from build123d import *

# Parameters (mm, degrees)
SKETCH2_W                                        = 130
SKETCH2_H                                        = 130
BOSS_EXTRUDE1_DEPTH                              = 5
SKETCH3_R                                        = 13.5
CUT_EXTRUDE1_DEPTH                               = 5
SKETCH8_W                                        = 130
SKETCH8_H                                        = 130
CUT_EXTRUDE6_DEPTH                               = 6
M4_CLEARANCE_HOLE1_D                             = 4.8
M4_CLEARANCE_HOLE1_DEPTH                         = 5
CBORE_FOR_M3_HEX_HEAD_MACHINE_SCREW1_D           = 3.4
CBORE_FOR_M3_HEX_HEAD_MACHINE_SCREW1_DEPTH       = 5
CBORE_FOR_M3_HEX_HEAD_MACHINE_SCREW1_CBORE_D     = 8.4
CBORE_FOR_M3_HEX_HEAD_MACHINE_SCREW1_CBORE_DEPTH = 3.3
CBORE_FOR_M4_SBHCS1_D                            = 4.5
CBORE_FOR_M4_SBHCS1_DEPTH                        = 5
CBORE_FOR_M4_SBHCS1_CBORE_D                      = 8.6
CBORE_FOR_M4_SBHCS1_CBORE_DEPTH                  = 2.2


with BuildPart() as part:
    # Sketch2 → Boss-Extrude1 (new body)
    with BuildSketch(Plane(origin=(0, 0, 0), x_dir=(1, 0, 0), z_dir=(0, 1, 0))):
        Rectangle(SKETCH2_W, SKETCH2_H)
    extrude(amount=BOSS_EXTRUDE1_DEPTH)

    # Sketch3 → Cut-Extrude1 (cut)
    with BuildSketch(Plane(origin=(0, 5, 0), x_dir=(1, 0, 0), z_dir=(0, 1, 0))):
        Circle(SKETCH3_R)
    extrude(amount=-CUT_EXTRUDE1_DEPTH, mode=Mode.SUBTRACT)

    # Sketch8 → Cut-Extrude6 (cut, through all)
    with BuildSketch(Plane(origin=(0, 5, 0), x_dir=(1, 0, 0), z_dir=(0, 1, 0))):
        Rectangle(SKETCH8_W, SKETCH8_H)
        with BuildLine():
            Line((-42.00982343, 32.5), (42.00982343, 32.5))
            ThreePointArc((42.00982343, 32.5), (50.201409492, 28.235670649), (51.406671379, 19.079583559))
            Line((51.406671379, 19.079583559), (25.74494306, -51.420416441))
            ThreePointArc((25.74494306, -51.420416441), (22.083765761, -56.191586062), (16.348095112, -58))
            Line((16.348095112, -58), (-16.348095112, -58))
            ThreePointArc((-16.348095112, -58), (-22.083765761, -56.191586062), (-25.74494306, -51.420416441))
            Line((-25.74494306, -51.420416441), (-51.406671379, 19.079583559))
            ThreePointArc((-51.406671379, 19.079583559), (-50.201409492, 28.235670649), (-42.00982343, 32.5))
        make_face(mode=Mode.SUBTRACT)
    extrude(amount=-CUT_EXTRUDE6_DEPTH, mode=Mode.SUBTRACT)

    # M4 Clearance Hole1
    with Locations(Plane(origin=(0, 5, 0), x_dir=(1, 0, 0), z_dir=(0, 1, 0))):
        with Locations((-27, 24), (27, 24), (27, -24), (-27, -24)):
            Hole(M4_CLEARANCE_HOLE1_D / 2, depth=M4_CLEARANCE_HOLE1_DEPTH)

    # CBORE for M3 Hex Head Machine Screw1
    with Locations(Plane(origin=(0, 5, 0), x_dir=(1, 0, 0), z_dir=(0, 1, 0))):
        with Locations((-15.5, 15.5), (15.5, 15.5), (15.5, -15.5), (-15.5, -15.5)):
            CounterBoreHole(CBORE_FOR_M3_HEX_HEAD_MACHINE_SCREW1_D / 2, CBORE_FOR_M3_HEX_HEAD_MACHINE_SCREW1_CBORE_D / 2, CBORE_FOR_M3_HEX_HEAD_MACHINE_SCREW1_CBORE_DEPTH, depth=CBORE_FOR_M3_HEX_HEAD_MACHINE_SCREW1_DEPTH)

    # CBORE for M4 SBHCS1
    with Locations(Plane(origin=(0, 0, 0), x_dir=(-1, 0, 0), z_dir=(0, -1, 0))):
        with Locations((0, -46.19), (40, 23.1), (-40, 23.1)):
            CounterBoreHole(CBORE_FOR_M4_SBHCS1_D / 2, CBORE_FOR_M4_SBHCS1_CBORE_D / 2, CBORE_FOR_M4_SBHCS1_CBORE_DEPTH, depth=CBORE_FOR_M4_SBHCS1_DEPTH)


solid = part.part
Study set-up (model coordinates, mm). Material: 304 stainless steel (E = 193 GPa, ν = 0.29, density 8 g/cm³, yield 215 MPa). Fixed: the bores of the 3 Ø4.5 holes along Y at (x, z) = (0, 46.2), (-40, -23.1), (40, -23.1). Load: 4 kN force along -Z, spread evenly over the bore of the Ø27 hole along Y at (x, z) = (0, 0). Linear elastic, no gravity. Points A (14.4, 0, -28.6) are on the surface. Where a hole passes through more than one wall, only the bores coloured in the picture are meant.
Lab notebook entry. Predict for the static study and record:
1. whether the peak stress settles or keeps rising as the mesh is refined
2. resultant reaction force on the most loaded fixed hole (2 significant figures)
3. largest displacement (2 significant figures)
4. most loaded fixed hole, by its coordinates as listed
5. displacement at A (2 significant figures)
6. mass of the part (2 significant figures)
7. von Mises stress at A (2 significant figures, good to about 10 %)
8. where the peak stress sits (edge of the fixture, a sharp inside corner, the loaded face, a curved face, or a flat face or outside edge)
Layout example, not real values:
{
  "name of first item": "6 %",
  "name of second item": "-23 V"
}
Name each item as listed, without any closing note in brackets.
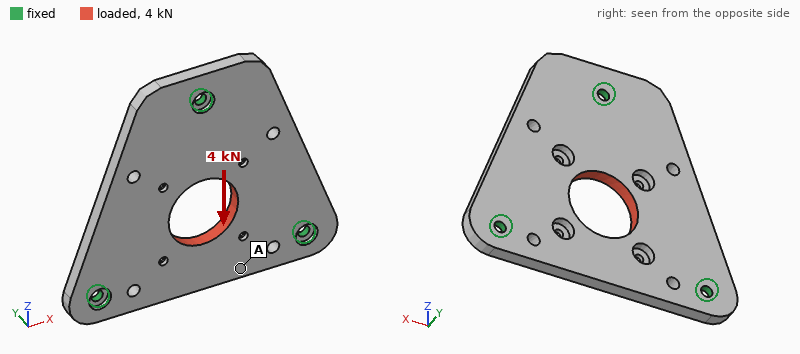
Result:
{
  "whether the peak stress settles or keeps rising as the mesh is refined": "keeps rising",
  "resultant reaction force on the most loaded fixed hole": "1.7 kN",
  "largest displacement": "7.1 µm",
  "most loaded fixed hole, by its coordinates as listed": "(0, 46.2)",
  "displacement at A": "5.4 µm",
  "mass of the part": "250 g",
  "von Mises stress at A": "9.4 MPa",
  "where the peak stress sits": "edge of the fixture"
}
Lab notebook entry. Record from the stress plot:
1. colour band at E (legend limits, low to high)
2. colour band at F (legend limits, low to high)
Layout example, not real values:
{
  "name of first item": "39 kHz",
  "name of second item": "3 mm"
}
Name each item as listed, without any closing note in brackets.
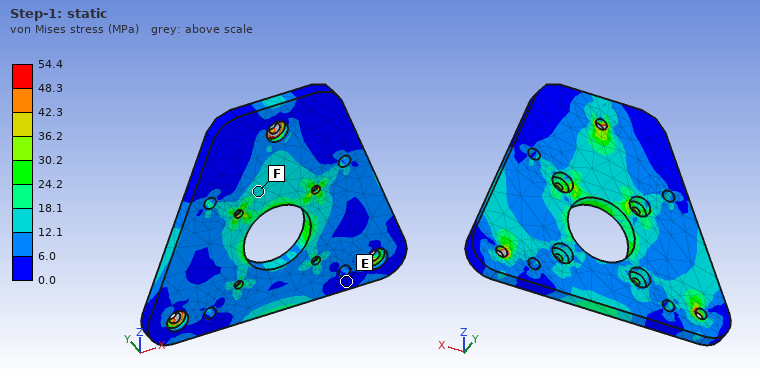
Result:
{
  "colour band at E": "0.0 to 6.0 MPa",
  "colour band at F": "12.1 to 18.1 MPa"
}
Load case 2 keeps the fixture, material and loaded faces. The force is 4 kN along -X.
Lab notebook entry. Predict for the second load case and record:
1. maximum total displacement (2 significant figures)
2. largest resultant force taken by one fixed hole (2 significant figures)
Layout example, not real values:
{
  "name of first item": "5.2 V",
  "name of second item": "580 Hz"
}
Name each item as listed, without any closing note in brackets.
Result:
{
  "maximum total displacement": "5.4 µm",
  "largest resultant force taken by one fixed hole": "1.4 kN"
}
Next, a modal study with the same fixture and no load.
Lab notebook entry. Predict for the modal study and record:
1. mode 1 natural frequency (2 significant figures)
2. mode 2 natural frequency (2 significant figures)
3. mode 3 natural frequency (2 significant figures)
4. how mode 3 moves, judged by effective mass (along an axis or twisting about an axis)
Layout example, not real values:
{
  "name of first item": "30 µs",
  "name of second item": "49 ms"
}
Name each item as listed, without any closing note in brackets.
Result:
{
  "mode 1 natural frequency": "2700 Hz",
  "mode 2 natural frequency": "2800 Hz",
  "mode 3 natural frequency": "3600 Hz",
  "how mode 3 moves, judged by effective mass": "twisting about X"
}
